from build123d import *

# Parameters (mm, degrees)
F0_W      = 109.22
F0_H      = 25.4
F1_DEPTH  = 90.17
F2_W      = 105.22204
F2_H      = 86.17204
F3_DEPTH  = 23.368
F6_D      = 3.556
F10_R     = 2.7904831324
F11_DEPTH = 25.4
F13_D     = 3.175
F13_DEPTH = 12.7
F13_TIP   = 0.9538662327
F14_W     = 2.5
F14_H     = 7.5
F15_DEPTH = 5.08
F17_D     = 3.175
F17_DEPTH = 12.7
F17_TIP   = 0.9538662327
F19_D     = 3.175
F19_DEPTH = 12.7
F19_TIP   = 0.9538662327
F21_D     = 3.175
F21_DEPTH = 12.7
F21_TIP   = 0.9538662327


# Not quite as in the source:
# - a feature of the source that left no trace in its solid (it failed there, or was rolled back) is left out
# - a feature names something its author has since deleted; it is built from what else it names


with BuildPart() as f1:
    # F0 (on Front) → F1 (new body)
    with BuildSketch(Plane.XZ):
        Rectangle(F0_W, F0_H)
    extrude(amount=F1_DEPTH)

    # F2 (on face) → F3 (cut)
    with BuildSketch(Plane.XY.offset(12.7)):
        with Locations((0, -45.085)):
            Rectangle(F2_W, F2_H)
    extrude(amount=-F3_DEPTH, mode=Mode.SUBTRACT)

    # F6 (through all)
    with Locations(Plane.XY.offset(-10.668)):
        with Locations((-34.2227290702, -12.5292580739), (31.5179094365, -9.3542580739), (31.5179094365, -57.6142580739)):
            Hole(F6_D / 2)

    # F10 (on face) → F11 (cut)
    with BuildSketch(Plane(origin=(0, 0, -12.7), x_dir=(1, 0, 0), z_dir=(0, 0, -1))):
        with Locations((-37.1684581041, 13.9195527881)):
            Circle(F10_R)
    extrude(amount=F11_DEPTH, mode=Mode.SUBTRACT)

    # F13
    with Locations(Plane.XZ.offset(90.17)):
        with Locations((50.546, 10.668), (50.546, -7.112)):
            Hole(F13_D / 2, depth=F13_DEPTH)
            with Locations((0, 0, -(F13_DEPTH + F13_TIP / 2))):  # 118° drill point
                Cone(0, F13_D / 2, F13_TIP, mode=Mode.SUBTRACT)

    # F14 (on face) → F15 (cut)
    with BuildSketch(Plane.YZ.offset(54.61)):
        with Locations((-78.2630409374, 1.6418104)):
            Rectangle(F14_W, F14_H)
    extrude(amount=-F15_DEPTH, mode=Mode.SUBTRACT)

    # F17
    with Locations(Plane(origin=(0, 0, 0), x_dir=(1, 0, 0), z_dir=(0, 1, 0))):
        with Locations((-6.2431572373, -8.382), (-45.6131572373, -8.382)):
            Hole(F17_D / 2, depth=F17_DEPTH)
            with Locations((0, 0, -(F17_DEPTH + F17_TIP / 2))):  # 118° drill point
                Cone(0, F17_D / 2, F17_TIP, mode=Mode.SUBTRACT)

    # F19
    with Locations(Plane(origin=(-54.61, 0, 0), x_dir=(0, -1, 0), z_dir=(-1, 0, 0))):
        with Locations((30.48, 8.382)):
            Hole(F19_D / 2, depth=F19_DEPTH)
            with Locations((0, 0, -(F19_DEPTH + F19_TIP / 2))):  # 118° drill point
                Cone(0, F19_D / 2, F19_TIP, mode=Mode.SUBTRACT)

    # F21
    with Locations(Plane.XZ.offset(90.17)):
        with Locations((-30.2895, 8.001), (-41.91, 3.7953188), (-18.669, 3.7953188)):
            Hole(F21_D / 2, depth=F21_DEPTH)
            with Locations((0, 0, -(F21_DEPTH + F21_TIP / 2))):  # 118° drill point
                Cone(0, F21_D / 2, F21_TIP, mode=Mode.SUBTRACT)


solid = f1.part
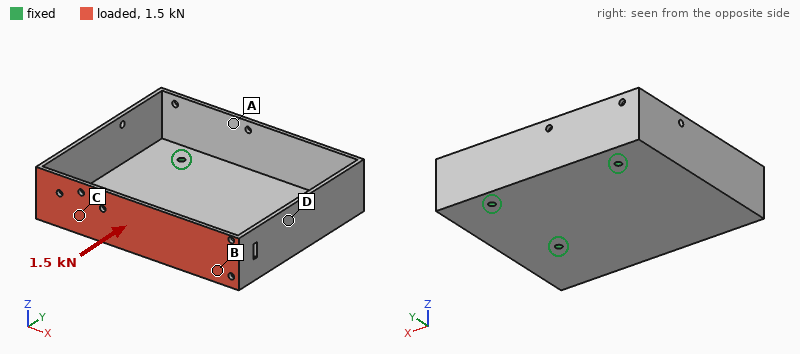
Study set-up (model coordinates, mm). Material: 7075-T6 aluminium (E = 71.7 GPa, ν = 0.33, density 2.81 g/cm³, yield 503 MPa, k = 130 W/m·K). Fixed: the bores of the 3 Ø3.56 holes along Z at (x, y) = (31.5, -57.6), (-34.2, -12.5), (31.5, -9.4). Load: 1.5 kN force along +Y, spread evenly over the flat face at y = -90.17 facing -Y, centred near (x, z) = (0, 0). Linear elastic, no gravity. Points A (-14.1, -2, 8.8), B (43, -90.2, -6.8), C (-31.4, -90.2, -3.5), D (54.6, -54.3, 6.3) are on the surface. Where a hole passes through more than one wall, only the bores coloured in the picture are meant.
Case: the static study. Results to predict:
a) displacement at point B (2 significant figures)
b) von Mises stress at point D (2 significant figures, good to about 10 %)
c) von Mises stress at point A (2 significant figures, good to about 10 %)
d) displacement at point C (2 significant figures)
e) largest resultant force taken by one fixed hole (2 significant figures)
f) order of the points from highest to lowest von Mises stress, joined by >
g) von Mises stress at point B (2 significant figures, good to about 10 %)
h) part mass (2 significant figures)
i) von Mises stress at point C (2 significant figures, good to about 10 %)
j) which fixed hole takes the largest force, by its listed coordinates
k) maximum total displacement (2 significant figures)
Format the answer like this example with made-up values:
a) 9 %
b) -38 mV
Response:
a) 0.32 mm
b) 50 MPa
c) 28 MPa
d) 1.4 mm
e) 740 N
f) B > C > D > A
g) 130 MPa
h) 110 g
i) 86 MPa
j) (-34.2, -12.5)
k) 1.7 mm
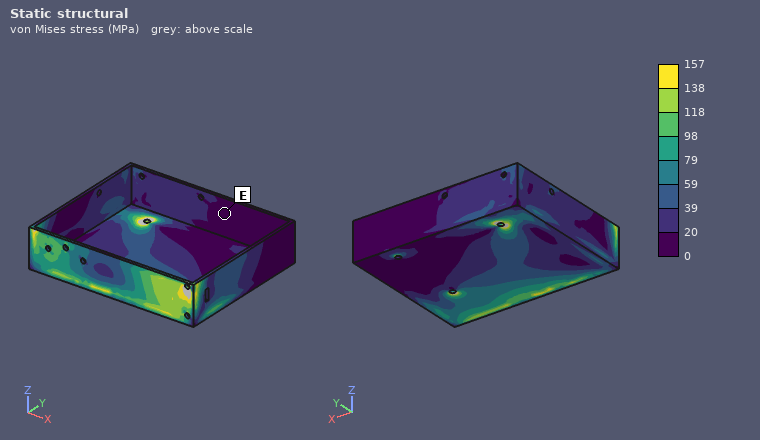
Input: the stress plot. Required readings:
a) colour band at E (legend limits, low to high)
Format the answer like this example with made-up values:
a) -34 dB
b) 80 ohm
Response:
a) 0 to 20 MPa
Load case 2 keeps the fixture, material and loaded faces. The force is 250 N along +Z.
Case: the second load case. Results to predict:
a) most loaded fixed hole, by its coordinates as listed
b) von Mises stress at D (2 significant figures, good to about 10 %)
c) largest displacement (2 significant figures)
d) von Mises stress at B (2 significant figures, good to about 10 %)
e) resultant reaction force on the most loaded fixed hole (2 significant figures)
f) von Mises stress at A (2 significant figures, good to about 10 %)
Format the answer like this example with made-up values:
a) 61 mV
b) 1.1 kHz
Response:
a) (31.5, -57.6)
b) 31 MPa
c) 1.6 mm
d) 40 MPa
e) 290 N
f) 25 MPa
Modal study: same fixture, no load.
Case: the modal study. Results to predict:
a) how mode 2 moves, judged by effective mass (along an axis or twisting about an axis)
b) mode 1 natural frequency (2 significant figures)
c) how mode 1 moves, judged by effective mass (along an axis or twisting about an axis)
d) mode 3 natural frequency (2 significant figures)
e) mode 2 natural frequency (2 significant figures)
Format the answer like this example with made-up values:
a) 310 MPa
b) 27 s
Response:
a) along Z
b) 370 Hz
c) along Z
d) 1800 Hz
e) 1000 Hz
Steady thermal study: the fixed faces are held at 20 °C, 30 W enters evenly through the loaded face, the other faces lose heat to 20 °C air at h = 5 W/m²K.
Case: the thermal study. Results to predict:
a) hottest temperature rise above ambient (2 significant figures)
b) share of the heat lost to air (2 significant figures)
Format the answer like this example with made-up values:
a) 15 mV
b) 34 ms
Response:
a) 58 K
b) 13 %
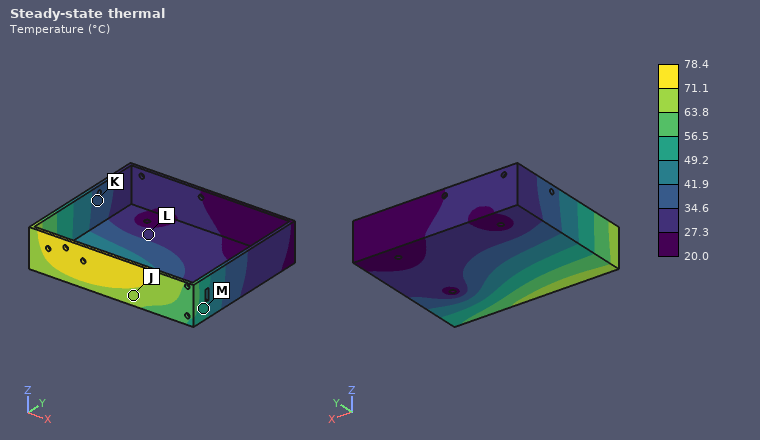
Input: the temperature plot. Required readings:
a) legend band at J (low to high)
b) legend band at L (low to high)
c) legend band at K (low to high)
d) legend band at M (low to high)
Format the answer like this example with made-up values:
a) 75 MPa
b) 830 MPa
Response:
a) 63.8 to 71.1 °C
b) 27.3 to 34.6 °C
c) 34.6 to 41.9 °C
d) 49.2 to 56.5 °C
